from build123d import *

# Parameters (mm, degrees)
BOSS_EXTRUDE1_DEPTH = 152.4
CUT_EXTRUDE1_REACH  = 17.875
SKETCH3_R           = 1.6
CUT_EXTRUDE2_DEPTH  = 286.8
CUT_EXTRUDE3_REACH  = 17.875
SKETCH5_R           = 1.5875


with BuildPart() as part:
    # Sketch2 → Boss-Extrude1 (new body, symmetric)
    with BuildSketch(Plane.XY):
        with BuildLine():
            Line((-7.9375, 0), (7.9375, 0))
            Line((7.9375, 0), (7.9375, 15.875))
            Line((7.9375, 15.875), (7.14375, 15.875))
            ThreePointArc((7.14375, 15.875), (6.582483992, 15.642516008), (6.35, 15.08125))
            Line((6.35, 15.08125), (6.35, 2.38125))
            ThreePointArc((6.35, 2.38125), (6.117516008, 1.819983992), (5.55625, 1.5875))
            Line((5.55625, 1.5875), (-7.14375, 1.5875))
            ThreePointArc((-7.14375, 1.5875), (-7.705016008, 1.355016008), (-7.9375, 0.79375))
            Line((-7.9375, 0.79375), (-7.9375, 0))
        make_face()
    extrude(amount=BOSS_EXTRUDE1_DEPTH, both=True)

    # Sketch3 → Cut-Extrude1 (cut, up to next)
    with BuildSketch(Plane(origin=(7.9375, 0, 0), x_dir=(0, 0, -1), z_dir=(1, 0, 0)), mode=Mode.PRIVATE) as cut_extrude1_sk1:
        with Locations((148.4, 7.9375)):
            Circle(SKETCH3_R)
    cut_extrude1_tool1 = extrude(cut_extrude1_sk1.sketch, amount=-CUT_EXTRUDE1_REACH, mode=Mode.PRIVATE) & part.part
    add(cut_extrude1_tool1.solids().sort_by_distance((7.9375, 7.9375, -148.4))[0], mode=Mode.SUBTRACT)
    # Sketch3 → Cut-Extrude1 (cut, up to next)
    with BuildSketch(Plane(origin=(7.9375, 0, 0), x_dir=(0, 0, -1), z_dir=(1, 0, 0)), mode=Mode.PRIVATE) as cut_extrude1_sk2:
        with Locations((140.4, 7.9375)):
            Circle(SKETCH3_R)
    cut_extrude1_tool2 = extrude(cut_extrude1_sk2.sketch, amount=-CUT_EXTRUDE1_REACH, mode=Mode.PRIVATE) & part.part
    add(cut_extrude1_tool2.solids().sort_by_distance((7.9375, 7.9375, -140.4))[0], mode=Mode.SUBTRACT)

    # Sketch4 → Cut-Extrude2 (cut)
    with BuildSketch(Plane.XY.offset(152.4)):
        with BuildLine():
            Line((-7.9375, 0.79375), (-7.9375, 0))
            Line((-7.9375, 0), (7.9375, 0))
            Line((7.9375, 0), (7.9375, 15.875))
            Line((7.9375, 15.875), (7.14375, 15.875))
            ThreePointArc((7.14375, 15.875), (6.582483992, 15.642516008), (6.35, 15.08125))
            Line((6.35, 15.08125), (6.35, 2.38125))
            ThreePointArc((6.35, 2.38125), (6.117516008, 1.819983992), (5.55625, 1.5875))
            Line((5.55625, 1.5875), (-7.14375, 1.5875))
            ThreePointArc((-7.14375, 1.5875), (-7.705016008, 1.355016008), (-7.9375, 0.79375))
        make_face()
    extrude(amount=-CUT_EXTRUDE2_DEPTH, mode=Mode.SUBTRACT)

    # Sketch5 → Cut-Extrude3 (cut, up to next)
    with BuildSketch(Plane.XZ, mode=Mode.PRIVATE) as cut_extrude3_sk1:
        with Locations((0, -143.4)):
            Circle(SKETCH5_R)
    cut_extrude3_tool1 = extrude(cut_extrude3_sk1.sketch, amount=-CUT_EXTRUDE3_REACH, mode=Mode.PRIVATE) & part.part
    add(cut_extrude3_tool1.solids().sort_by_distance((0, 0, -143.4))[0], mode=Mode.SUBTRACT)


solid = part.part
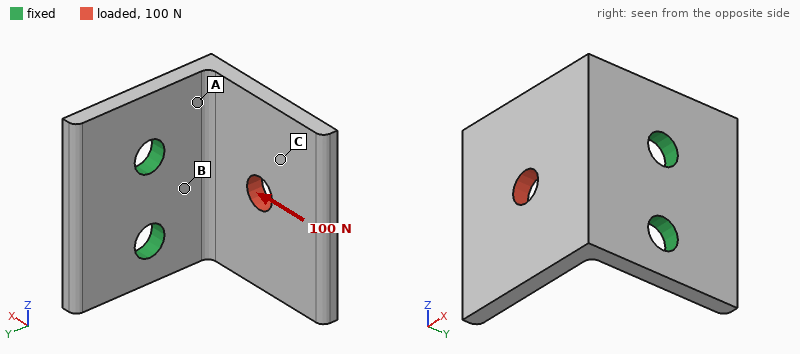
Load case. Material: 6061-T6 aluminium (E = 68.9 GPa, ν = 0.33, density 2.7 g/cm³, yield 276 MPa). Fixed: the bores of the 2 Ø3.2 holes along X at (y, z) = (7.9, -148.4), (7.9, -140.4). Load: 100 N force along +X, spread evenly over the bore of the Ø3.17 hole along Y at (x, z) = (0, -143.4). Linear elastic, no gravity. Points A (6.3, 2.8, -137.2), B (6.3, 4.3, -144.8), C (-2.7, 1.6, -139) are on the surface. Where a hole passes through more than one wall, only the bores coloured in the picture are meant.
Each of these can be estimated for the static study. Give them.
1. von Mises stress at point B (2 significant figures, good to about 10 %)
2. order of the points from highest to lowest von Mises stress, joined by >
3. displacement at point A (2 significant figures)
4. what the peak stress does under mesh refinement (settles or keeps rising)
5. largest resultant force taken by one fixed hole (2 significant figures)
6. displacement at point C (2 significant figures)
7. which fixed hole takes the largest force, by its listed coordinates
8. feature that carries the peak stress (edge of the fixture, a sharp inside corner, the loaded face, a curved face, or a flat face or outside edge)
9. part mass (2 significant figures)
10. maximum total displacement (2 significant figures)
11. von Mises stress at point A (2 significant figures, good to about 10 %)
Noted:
40 MPa
B > A > C
12 µm
keeps rising
58 N
47 µm
(7.9, -140.4)
edge of the fixture
2.2 g
72 µm
24 MPa
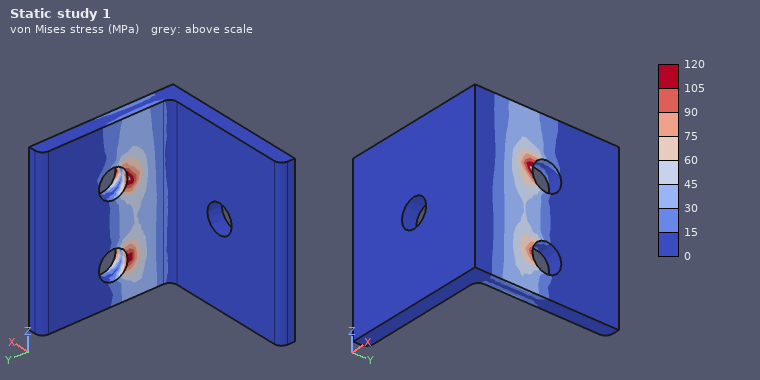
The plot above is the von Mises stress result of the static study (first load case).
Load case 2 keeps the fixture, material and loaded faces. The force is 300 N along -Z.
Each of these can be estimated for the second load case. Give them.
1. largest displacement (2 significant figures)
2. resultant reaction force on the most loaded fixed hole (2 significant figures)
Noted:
0.14 mm
310 N
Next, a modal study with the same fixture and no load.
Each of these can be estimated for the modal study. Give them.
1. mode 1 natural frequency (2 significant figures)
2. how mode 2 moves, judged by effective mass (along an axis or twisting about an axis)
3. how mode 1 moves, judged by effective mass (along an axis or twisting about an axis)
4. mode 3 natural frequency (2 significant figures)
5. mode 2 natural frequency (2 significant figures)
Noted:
3700 Hz
along Z
along Y
12 kHz
7400 Hz
